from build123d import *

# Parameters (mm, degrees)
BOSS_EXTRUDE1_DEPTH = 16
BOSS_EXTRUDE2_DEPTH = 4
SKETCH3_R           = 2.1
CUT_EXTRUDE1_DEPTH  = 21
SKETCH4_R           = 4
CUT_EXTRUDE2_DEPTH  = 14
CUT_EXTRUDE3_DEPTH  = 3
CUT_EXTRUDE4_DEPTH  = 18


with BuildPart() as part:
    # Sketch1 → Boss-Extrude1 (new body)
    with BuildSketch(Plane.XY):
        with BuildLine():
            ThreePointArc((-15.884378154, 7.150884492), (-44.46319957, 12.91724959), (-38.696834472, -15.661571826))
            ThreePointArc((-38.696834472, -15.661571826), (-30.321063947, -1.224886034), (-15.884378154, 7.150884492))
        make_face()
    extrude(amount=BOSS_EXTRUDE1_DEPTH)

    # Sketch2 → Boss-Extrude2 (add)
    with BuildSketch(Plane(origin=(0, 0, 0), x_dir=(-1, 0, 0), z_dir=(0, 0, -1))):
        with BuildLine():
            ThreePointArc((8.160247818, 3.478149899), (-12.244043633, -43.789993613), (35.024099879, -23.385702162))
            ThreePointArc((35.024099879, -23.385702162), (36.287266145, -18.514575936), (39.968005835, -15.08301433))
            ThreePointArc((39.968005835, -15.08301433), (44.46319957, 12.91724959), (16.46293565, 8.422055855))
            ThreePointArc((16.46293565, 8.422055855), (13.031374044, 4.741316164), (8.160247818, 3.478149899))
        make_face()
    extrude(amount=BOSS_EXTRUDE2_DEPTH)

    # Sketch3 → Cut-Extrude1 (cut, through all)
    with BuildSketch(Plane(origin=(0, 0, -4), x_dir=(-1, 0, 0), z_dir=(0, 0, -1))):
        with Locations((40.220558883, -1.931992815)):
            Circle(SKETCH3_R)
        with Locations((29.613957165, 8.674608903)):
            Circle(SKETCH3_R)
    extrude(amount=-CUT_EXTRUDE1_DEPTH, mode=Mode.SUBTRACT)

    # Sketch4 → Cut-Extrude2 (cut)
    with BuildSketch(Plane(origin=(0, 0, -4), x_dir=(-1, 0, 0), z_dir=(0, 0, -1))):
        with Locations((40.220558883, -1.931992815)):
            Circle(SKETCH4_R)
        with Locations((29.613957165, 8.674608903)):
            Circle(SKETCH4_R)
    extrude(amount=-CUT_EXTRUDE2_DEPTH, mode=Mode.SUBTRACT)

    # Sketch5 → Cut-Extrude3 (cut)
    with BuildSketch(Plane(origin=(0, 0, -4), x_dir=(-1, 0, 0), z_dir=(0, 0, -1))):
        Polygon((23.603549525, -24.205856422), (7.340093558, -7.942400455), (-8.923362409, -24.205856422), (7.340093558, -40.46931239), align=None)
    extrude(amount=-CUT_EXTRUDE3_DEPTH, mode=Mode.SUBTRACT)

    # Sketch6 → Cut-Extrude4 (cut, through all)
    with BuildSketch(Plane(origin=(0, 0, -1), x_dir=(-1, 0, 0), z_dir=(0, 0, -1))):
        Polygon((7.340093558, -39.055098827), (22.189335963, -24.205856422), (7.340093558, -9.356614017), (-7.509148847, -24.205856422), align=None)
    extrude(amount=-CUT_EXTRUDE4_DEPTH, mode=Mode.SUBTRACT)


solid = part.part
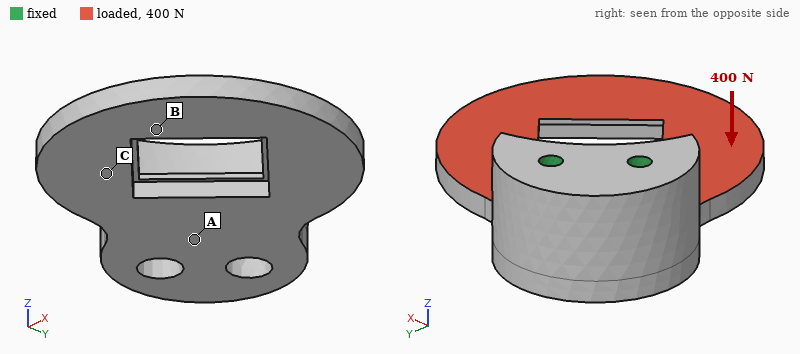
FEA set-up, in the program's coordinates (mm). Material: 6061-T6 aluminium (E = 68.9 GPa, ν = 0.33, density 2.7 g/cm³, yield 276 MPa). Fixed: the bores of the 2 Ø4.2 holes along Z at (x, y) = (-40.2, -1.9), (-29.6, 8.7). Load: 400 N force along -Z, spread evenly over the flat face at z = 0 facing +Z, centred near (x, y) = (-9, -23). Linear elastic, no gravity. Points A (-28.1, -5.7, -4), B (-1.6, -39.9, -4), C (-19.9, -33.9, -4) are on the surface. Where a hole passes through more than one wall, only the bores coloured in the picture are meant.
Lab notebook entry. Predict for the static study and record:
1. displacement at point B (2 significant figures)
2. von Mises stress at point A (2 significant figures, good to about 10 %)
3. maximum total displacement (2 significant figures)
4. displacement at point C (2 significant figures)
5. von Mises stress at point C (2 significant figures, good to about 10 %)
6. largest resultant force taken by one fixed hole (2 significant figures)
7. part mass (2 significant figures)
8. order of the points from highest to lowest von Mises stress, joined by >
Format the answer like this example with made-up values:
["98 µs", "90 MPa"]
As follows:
["0.77 mm", "84 MPa", "1.0 mm", "0.39 mm", "37 MPa", "200 N", "52 g", "A > C > B"]
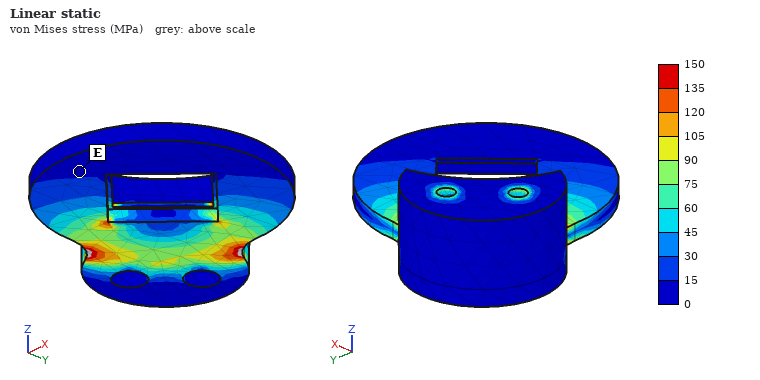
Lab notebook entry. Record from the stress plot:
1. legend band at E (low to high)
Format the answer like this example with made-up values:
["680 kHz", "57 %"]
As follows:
["0 to 15 MPa"]
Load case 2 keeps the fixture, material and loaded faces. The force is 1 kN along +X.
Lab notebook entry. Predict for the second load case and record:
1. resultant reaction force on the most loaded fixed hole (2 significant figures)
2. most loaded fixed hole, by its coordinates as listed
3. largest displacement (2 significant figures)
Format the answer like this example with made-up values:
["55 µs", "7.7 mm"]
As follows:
["1.8 kN", "(-40.2, -1.9)", "0.17 mm"]
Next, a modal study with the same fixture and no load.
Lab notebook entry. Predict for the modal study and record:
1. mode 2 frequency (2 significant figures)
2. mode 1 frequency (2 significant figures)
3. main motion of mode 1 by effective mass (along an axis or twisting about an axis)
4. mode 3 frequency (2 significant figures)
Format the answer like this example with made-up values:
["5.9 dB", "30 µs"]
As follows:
["2100 Hz", "830 Hz", "along Z", "3100 Hz"]
